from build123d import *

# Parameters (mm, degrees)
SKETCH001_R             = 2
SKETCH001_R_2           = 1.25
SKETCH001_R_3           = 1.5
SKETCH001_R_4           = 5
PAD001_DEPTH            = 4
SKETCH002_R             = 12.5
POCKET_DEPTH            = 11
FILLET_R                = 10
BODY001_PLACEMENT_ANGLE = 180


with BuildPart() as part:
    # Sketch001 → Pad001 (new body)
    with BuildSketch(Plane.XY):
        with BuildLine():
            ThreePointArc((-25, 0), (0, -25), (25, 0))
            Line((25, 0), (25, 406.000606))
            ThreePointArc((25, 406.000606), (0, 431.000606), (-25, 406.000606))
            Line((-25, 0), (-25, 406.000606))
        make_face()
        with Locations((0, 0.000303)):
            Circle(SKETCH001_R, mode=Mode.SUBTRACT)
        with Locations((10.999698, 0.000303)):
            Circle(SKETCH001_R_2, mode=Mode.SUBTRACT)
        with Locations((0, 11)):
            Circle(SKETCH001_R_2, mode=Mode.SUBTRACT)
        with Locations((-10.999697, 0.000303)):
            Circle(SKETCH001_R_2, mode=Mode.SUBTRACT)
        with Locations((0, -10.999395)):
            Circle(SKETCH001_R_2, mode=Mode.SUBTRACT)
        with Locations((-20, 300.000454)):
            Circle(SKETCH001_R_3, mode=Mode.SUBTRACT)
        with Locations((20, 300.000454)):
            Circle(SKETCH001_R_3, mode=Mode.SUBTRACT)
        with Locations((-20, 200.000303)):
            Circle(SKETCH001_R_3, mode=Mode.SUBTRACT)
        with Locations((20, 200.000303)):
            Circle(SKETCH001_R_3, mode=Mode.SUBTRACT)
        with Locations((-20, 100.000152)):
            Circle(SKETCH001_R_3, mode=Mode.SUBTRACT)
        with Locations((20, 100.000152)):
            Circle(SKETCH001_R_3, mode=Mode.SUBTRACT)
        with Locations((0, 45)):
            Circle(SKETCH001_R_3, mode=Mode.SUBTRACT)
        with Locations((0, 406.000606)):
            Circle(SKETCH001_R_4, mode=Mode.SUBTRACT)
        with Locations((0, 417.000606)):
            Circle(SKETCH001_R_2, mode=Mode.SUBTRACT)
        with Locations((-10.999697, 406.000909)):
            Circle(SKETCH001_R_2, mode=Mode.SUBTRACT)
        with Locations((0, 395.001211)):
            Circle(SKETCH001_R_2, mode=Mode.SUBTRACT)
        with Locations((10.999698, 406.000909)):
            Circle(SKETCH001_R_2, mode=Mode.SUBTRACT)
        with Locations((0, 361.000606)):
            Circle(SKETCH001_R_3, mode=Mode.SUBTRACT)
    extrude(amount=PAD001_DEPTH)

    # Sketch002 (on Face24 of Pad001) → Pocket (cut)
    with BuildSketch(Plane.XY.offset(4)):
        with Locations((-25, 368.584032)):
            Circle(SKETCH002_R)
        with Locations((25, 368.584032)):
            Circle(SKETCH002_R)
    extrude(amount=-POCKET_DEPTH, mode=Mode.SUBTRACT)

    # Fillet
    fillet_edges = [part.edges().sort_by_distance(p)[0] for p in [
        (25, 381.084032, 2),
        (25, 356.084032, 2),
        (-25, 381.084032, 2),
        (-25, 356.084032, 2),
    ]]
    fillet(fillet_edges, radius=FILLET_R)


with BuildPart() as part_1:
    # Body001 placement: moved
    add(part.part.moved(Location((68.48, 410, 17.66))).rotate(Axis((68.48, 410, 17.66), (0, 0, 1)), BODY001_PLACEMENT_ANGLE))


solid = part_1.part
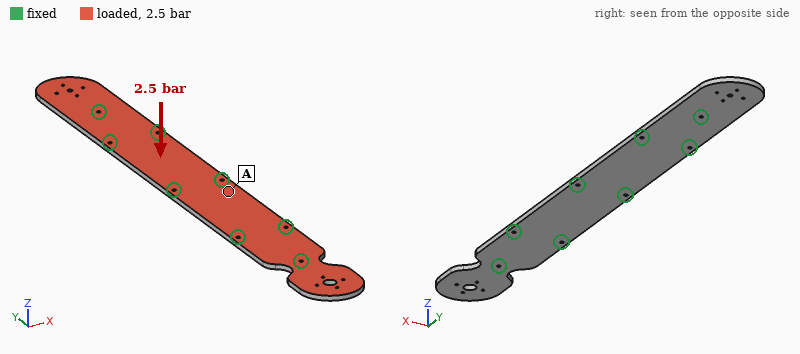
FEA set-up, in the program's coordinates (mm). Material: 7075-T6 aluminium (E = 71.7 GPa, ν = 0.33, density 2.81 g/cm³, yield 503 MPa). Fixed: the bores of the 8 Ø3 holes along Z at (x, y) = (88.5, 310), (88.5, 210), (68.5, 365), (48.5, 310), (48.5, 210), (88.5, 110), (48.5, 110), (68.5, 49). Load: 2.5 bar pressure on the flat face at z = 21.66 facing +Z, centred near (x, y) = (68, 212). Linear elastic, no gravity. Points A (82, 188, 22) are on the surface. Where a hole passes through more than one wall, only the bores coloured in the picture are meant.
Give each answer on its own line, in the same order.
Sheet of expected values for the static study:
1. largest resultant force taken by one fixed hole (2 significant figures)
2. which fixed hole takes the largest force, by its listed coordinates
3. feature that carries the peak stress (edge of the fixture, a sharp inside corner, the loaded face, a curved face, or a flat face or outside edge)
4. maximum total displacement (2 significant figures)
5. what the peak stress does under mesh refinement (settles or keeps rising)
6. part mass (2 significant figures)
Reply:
1.3 kN
(68.5, 365)
edge of the fixture
2.7 mm
keeps rising
240 g
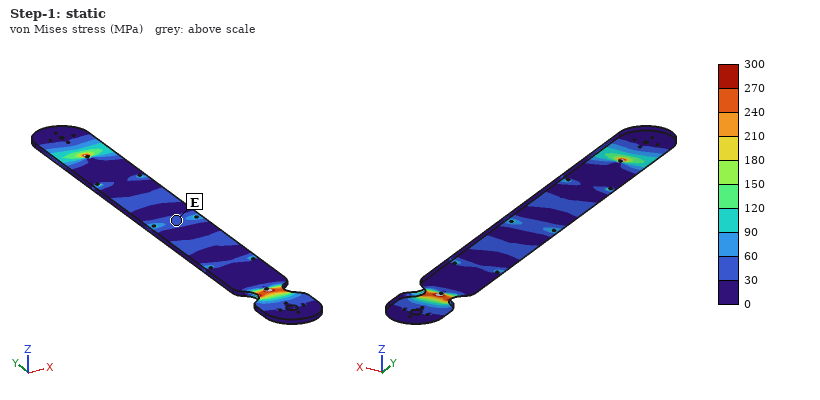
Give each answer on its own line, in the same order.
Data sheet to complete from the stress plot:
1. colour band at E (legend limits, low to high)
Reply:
30 to 60 MPa
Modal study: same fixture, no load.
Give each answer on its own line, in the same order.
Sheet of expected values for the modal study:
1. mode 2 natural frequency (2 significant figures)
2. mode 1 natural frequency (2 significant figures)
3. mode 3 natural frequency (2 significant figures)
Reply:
700 Hz
580 Hz
1600 Hz
